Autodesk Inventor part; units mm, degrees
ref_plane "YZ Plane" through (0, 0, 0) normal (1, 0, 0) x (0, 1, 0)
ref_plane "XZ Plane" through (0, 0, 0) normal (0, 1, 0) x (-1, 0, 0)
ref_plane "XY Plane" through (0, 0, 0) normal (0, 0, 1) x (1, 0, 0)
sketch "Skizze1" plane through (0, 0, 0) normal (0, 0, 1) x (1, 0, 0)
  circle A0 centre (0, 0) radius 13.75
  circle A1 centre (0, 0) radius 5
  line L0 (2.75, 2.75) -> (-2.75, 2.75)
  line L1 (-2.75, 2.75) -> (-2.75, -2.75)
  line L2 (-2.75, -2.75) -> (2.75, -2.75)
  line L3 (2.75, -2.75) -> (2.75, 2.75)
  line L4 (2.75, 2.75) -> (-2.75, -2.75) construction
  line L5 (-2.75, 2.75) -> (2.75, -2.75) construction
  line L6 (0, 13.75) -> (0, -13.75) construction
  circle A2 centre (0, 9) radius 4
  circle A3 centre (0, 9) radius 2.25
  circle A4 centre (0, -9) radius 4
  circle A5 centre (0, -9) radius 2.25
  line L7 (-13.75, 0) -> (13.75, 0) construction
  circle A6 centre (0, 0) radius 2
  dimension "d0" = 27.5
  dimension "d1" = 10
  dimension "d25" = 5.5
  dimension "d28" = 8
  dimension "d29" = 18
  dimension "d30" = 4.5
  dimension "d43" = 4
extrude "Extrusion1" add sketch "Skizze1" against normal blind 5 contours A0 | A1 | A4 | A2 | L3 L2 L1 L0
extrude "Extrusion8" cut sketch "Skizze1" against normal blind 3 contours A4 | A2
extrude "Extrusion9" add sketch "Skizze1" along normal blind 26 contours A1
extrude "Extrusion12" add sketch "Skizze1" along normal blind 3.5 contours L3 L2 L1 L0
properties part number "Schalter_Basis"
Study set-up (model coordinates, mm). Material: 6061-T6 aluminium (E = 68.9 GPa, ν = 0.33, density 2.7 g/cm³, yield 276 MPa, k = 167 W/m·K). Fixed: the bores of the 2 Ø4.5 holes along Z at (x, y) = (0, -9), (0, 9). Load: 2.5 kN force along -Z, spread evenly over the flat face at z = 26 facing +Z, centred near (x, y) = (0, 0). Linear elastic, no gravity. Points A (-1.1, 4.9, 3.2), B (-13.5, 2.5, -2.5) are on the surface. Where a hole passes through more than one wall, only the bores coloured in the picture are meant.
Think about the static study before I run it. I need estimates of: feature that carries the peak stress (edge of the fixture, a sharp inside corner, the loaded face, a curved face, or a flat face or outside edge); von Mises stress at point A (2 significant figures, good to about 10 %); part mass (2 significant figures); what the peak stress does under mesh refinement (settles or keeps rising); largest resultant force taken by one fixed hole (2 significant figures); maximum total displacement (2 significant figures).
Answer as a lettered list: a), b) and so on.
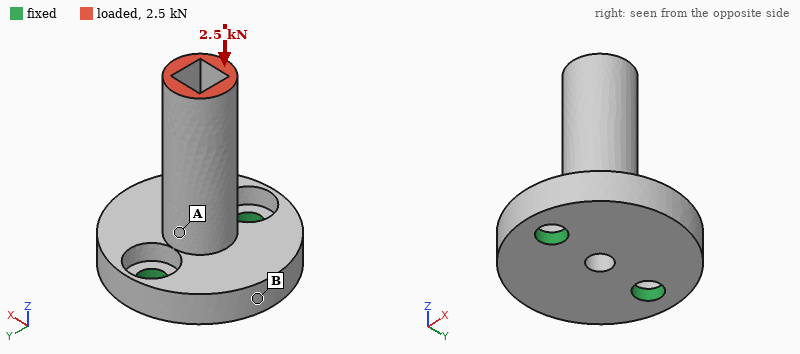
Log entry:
a) edge of the fixture
b) 47 MPa
c) 10 g
d) keeps rising
e) 1.4 kN
f) 33 µm
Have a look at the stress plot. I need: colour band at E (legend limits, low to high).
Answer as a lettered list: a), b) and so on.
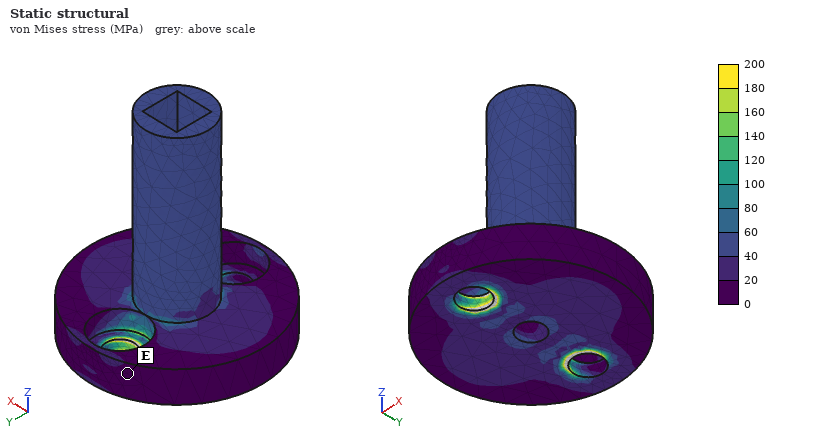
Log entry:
a) 0 to 20 MPa
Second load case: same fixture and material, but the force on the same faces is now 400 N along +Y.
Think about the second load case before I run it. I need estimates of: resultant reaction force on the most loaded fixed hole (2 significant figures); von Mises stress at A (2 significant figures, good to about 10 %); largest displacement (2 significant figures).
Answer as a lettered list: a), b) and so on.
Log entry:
a) 810 N
b) 100 MPa
c) 0.15 mm
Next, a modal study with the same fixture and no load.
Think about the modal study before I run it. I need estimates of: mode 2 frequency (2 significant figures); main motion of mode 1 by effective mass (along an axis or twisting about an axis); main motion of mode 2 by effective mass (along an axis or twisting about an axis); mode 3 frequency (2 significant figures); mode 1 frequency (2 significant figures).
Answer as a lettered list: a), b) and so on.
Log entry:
a) 8300 Hz
b) along X
c) along Y
d) 19 kHz
e) 5200 Hz
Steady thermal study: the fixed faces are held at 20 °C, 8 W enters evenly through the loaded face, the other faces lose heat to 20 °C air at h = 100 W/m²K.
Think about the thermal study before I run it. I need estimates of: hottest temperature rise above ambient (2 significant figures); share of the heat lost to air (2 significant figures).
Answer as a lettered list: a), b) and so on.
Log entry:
a) 25 K
b) 26 %
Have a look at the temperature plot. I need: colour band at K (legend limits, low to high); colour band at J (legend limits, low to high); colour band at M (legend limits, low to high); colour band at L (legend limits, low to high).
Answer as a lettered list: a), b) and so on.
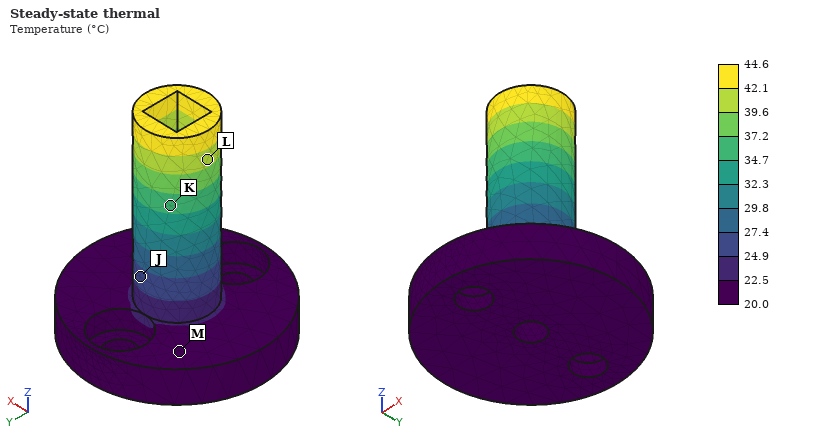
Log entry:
a) 34.7 to 37.2 °C
b) 24.9 to 27.4 °C
c) 20.0 to 22.5 °C
d) 39.6 to 42.1 °C
